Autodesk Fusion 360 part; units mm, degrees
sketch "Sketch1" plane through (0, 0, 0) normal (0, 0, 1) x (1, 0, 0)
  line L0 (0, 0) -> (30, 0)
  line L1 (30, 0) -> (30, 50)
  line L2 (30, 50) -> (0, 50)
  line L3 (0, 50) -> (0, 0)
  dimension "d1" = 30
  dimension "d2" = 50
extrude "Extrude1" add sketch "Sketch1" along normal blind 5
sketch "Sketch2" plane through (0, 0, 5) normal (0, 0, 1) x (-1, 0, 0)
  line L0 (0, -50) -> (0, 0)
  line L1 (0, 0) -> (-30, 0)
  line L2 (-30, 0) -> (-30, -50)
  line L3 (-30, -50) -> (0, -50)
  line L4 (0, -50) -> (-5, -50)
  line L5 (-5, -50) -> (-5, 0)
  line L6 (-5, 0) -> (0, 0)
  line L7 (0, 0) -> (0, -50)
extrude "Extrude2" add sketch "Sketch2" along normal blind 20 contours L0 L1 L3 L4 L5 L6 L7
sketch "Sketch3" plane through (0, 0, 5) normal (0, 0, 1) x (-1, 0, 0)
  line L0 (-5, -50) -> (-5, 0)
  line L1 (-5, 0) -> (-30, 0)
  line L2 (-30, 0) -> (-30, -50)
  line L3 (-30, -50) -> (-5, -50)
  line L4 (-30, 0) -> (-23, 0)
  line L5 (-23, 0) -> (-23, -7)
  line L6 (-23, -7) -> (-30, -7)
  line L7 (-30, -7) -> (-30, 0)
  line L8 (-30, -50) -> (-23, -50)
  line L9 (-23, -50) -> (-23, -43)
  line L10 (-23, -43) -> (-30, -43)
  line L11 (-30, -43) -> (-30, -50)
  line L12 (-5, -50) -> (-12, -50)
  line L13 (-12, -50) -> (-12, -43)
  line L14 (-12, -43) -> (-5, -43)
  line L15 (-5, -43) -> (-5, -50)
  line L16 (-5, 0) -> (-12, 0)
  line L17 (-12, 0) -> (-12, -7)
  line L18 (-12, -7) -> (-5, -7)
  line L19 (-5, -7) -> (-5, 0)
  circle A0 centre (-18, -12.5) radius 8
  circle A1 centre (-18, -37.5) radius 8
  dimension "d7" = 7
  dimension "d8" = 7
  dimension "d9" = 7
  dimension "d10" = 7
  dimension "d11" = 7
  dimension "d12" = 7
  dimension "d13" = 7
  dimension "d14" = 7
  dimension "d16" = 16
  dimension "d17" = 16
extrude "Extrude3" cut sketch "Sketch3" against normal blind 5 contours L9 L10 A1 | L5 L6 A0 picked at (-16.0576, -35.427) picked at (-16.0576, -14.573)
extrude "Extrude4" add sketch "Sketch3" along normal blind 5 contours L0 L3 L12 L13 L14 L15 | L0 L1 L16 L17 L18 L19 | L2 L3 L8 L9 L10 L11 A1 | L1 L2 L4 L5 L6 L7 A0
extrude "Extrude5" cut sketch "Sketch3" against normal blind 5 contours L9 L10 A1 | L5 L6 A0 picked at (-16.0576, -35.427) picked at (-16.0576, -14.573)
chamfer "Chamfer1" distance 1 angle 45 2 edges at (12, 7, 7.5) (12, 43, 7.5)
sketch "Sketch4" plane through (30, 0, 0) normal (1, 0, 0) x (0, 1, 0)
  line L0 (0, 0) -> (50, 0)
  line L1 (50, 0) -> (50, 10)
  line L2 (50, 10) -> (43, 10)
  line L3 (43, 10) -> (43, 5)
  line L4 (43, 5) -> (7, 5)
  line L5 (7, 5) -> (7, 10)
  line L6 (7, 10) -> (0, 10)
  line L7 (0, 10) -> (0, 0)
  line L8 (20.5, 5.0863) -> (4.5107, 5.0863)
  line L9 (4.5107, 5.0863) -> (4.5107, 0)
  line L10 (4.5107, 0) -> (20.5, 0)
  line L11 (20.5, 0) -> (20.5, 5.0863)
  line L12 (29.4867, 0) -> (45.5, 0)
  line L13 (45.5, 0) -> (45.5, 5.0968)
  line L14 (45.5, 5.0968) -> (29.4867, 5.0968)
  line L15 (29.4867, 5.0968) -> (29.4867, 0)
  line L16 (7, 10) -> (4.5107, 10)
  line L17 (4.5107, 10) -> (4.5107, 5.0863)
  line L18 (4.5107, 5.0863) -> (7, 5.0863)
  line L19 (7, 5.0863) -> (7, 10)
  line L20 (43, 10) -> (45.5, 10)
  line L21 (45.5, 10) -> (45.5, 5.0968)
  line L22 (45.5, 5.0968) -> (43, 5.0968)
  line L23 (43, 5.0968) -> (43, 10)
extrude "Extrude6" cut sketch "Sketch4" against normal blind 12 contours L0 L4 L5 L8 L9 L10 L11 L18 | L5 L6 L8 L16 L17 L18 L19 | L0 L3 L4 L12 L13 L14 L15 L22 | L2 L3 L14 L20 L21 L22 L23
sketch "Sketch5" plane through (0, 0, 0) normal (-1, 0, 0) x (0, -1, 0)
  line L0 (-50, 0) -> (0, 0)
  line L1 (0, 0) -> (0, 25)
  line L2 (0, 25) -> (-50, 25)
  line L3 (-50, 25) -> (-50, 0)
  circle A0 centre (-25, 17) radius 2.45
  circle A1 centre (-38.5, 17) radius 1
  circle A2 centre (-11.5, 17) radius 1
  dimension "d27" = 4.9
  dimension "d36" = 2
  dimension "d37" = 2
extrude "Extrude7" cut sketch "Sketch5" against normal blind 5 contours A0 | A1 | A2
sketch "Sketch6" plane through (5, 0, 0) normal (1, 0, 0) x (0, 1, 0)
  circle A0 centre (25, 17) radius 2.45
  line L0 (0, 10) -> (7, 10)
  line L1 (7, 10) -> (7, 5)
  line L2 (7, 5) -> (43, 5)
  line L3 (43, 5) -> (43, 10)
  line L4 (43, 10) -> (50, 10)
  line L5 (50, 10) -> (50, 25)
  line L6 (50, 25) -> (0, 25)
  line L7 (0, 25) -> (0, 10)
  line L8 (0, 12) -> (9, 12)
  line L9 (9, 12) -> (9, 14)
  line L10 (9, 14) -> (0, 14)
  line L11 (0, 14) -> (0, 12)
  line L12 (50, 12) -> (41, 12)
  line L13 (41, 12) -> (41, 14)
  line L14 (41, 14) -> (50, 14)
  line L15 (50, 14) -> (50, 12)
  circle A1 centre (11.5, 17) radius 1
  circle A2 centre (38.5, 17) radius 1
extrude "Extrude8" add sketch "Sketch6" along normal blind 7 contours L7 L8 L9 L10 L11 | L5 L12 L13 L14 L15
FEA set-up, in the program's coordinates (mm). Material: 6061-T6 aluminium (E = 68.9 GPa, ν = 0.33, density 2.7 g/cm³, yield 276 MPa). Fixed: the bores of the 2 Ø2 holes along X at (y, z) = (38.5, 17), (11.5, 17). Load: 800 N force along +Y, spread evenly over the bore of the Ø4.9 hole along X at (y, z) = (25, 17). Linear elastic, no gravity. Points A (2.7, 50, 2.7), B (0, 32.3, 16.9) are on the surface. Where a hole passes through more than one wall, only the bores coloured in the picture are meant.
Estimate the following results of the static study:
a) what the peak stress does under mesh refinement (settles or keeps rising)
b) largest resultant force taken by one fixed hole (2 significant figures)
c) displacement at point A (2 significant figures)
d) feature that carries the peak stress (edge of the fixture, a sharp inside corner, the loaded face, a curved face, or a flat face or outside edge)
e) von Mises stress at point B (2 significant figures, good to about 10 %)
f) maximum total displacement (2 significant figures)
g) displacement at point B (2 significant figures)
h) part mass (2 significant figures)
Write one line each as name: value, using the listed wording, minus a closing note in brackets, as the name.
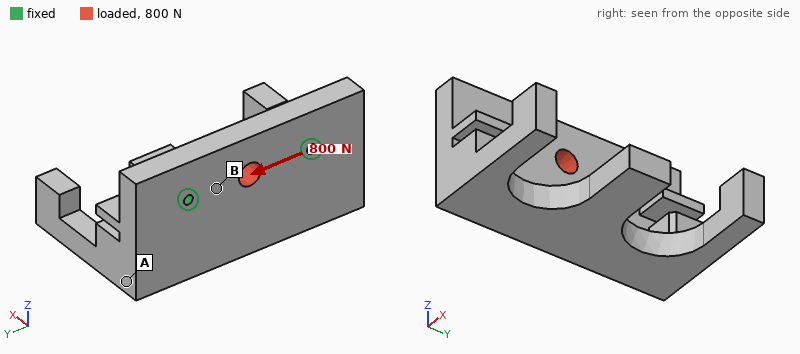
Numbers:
what the peak stress does under mesh refinement: keeps rising
largest resultant force taken by one fixed hole: 400 N
displacement at point A: 0.74 µm
feature that carries the peak stress: edge of the fixture
von Mises stress at point B: 9.6 MPa
maximum total displacement: 1.7 µm
displacement at point B: 0.86 µm
part mass: 28 g
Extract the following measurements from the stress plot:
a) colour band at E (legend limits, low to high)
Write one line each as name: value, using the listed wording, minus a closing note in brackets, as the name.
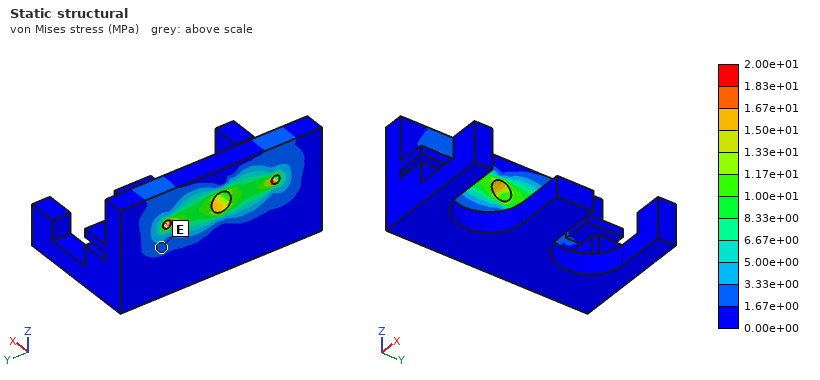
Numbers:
colour band at E: 1.67e+00 to 3.33e+00 MPa
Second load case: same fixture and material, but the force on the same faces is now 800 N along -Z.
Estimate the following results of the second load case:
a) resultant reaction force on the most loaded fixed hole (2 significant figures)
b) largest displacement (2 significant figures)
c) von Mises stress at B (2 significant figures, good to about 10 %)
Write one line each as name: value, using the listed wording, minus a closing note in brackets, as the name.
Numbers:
resultant reaction force on the most loaded fixed hole: 400 N
largest displacement: 3.5 µm
von Mises stress at B: 6.4 MPa
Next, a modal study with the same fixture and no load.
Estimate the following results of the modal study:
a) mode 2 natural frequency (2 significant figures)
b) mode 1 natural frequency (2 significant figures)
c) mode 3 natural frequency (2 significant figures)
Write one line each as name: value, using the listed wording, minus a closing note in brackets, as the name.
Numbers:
mode 2 natural frequency: 4500 Hz
mode 1 natural frequency: 3500 Hz
mode 3 natural frequency: 6300 Hz
